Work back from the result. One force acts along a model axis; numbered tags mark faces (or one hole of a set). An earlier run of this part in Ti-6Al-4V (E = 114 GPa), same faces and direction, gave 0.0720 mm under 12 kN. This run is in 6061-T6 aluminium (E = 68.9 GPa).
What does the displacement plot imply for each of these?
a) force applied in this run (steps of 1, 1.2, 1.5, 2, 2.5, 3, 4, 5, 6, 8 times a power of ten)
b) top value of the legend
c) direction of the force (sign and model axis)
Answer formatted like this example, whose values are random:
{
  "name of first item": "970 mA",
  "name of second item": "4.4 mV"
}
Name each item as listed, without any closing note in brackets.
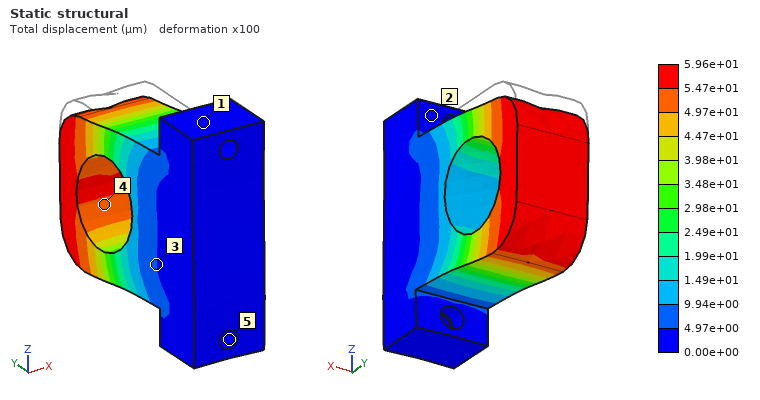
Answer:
{
  "force applied in this run": "6 kN",
  "top value of the legend": "5.96e+01 µm",
  "direction of the force": "-Z"
}
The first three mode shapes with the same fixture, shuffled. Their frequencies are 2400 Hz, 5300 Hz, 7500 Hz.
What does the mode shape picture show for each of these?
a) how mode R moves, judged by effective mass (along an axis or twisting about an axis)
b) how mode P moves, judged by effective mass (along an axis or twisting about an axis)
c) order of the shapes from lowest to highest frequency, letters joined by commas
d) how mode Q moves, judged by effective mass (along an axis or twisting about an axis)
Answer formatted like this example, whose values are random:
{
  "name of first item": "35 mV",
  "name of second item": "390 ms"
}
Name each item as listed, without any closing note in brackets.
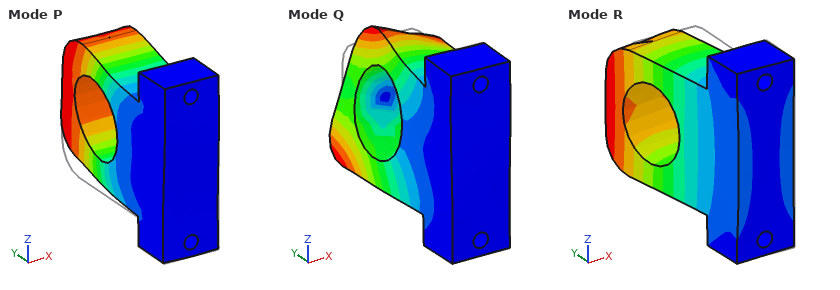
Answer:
{
  "how mode R moves, judged by effective mass": "along X",
  "how mode P moves, judged by effective mass": "along Z",
  "order of the shapes from lowest to highest frequency, letters joined by commas": "R, P, Q",
  "how mode Q moves, judged by effective mass": "twisting about Y"
}
